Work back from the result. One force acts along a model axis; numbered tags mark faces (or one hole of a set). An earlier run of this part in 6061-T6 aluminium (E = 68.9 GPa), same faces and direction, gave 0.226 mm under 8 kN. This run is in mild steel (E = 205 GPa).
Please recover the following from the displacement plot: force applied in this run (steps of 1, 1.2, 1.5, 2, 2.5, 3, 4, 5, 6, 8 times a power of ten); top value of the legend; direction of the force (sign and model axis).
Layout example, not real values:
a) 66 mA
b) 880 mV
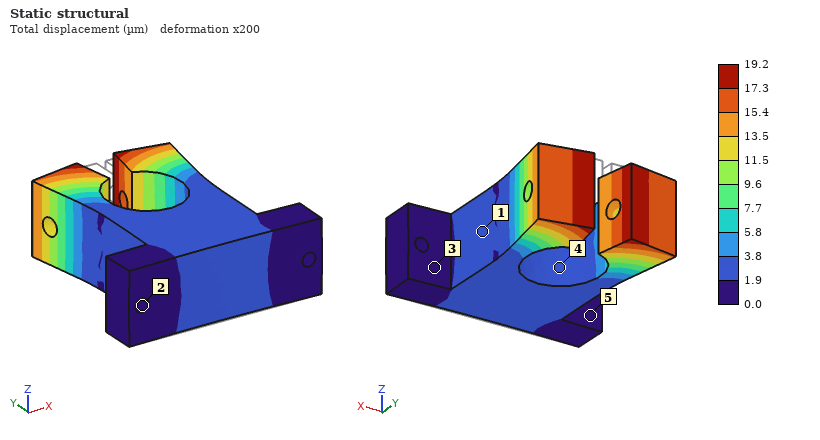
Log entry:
a) 2 kN
b) 19.2 µm
c) +Y
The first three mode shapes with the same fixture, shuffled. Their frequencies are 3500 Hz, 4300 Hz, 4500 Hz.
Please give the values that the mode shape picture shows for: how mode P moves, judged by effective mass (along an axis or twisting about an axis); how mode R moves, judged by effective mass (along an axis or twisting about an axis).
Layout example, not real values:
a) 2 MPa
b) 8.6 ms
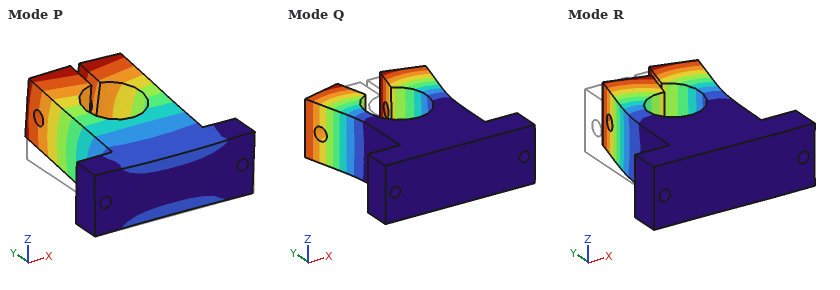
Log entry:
a) along Z
b) along X
